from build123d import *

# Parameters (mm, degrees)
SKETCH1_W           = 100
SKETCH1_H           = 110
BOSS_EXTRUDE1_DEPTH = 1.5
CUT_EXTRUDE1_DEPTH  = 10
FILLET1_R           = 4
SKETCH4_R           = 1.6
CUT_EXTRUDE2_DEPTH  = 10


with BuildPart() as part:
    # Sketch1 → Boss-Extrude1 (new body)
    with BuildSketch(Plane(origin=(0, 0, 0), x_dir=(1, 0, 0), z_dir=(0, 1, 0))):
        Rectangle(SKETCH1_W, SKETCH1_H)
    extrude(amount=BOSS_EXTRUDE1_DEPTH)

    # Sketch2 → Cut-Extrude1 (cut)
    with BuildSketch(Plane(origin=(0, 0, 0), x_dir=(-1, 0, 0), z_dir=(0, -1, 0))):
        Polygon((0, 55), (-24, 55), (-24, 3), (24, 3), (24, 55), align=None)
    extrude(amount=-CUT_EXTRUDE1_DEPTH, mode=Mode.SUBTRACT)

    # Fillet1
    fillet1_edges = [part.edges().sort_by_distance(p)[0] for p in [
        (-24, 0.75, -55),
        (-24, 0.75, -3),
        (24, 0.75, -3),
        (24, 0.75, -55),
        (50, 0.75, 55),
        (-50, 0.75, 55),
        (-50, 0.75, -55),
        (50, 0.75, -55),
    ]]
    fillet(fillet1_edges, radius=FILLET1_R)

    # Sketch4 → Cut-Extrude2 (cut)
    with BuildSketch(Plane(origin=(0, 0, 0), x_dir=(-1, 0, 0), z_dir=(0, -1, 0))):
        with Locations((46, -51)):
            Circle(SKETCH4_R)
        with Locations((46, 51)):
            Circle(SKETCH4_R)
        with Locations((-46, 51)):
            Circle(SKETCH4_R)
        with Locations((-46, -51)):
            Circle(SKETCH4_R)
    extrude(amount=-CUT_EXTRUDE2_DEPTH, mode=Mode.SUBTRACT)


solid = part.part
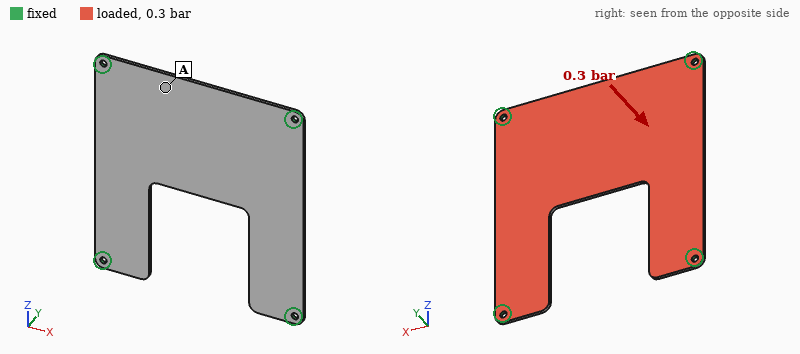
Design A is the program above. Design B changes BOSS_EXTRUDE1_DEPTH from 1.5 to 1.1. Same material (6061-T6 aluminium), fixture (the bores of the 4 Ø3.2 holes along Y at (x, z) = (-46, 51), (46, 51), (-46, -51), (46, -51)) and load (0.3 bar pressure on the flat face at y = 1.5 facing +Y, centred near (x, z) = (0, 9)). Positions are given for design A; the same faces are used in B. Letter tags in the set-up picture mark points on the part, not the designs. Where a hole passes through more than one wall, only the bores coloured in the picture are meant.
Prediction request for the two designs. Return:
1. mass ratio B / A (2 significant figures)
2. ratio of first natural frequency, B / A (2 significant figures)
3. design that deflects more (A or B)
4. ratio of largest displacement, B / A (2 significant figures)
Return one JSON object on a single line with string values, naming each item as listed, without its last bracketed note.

{"mass ratio B / A": "0.73", "ratio of first natural frequency, B / A": "0.74", "design that deflects more": "B", "ratio of largest displacement, B / A": "2.5"}
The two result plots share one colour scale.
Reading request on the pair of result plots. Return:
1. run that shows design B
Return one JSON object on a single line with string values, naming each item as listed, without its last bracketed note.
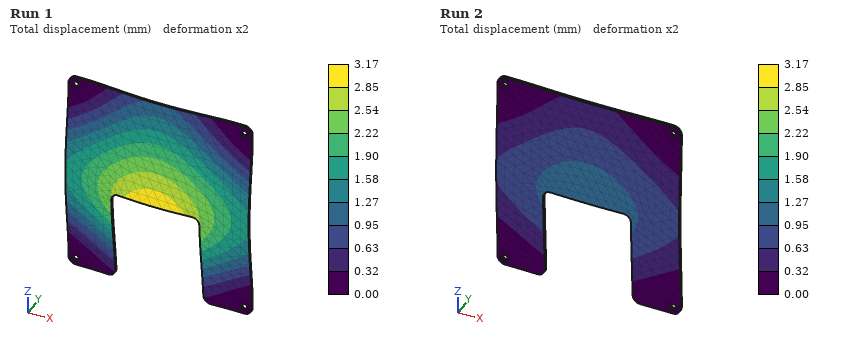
{"run that shows design B": "Run 1"}
